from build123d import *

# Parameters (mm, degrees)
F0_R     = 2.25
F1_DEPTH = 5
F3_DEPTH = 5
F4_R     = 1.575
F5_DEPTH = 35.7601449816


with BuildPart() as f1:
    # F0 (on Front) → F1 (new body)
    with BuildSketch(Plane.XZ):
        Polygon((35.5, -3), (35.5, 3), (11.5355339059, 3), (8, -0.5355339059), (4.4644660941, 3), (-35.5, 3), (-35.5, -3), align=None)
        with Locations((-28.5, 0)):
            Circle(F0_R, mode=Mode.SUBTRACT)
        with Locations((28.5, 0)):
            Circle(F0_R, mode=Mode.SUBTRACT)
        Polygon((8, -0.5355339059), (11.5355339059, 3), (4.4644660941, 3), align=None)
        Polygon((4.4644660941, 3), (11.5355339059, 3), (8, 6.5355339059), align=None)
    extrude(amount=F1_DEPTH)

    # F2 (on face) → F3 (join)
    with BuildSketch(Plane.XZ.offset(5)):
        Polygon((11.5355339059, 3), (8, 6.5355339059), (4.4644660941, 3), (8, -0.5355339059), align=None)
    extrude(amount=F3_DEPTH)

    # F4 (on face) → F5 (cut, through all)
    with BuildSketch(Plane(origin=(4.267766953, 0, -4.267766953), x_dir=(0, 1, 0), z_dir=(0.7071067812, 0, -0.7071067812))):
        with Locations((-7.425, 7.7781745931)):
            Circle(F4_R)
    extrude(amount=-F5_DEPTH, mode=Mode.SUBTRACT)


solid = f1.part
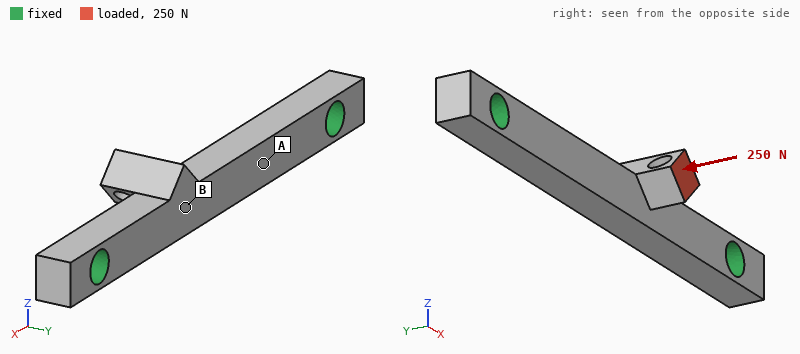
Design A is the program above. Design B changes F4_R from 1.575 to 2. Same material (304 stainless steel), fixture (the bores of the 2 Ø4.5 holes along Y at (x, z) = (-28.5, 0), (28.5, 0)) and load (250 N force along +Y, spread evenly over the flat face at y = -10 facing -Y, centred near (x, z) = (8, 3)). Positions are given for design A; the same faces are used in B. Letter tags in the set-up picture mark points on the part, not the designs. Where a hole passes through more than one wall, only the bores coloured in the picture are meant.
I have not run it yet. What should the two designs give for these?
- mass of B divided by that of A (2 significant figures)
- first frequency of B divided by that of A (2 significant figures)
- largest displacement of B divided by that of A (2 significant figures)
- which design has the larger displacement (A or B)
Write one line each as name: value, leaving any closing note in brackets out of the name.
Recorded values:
mass of B divided by that of A: 0.99
first frequency of B divided by that of A: 1.0
largest displacement of B divided by that of A: 1.1
which design has the larger displacement: B
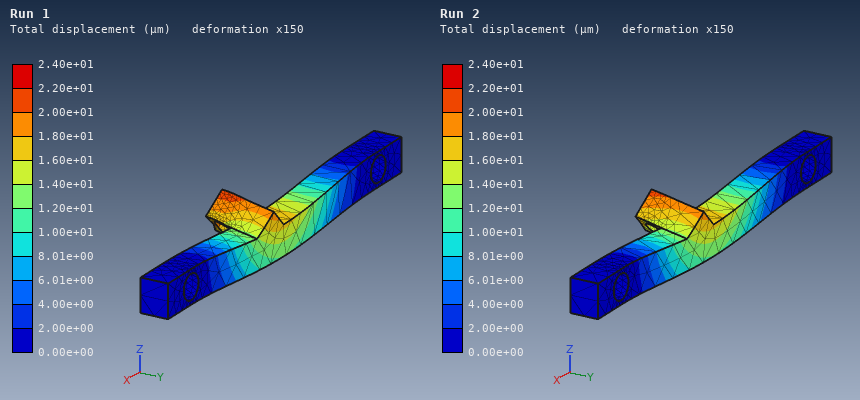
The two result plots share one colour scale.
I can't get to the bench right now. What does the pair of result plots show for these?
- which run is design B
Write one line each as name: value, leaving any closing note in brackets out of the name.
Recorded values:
which run is design B: Run 1
